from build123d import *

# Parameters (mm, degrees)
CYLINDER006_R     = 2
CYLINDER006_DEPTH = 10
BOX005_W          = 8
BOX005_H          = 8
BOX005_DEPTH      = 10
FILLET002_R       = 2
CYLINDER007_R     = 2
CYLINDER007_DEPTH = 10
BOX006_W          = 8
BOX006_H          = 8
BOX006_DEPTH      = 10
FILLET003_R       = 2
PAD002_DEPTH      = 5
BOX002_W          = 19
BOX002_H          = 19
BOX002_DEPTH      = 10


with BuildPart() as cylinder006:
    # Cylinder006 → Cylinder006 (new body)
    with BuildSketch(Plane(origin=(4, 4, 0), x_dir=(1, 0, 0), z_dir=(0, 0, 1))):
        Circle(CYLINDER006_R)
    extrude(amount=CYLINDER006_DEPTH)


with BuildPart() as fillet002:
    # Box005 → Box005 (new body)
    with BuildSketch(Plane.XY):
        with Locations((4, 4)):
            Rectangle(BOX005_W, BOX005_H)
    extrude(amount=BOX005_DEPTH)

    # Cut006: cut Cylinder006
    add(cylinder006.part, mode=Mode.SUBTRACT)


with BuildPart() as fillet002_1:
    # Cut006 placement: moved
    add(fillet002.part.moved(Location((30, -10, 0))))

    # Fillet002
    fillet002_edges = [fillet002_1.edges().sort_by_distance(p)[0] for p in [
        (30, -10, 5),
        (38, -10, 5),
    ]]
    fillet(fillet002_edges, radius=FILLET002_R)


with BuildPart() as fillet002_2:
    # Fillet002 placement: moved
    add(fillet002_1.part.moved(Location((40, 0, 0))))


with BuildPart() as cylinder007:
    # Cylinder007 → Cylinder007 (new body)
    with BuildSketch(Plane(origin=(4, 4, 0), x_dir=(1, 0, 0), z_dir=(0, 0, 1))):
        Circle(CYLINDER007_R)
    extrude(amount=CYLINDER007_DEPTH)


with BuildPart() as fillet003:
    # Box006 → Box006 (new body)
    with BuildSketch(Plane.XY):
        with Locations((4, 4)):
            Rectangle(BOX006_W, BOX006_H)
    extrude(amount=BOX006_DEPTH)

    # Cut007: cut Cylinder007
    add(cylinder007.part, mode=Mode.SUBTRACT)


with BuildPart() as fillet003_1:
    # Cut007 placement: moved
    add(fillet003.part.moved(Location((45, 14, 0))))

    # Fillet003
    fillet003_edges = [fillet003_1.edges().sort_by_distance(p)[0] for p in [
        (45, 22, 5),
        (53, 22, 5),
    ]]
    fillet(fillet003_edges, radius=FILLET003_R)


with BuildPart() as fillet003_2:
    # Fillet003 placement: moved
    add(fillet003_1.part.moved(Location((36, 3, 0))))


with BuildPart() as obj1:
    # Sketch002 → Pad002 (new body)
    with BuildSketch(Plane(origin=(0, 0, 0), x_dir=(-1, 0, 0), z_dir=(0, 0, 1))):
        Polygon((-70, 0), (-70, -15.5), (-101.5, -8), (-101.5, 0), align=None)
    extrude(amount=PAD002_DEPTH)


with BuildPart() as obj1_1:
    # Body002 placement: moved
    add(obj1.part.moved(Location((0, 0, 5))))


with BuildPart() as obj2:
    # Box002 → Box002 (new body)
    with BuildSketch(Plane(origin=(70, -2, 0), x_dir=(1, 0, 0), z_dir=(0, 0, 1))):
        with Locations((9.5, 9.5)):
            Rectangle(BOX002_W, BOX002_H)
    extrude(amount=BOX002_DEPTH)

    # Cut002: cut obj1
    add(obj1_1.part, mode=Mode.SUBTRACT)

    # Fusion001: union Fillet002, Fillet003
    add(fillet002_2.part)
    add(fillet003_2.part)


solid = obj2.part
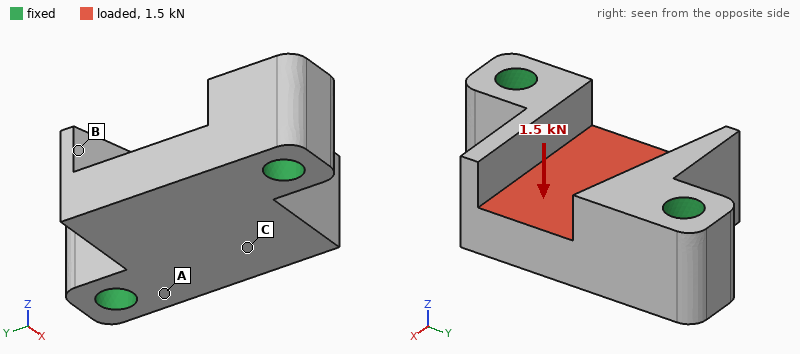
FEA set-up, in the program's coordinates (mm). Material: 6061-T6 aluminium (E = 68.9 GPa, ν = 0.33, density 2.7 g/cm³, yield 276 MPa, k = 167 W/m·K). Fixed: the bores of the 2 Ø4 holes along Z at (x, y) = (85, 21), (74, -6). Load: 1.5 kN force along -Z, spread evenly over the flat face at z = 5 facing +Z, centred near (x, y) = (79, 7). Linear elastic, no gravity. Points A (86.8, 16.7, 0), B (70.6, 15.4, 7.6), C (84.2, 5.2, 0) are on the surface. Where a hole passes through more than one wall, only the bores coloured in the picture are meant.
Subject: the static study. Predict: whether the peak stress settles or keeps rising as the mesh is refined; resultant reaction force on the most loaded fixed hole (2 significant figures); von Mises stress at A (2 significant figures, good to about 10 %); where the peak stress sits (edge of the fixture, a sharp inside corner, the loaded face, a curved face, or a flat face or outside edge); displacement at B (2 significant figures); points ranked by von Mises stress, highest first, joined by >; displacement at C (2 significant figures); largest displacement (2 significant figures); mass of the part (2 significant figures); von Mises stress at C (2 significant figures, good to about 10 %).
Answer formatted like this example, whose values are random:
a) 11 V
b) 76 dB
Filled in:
a) keeps rising
b) 820 N
c) 19 MPa
d) edge of the fixture
e) 12 µm
f) C > A > B
g) 9.0 µm
h) 14 µm
i) 9.0 g
j) 30 MPa
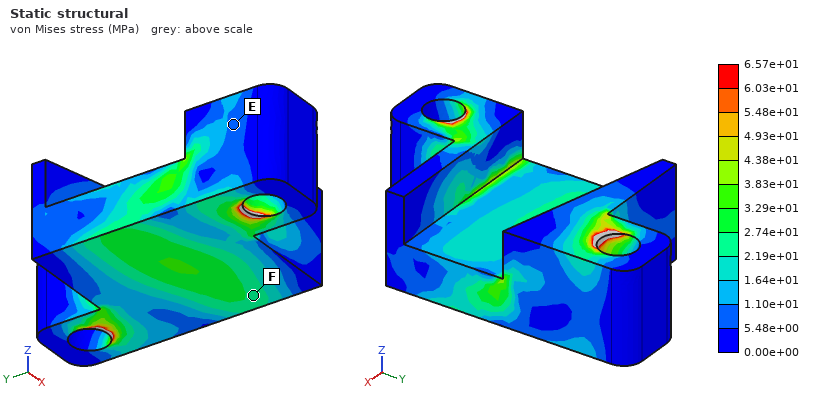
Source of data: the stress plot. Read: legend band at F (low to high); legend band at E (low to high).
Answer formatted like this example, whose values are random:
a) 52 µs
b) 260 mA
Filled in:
a) 2.19e+01 to 2.74e+01 MPa
b) 5.48e+00 to 1.10e+01 MPa
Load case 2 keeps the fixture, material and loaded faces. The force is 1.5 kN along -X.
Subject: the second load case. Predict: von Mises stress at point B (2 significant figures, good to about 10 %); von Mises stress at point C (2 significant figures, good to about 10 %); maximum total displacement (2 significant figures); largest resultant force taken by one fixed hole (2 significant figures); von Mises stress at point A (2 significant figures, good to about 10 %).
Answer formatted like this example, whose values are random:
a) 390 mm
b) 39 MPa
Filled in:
a) 5.2 MPa
b) 10 MPa
c) 7.9 µm
d) 790 N
e) 13 MPa
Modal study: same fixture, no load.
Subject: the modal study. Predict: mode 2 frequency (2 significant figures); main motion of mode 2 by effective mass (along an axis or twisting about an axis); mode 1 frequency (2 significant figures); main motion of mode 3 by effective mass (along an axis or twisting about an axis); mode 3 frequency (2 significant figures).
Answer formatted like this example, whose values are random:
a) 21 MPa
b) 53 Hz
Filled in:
a) 28 kHz
b) along Z
c) 24 kHz
d) along X
e) 37 kHz
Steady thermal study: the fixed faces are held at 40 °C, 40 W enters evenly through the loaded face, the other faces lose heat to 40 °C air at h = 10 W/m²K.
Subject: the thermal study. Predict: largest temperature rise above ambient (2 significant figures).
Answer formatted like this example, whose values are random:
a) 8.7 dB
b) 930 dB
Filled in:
a) 19 K
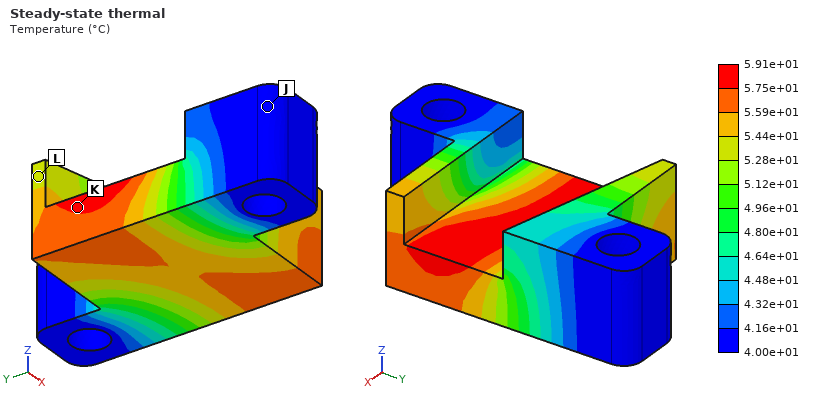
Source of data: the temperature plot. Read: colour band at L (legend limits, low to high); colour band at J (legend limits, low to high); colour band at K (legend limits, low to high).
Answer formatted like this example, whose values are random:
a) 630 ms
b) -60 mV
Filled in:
a) 5.28e+01 to 5.44e+01 °C
b) 4.00e+01 to 4.16e+01 °C
c) 5.75e+01 to 5.91e+01 °C
